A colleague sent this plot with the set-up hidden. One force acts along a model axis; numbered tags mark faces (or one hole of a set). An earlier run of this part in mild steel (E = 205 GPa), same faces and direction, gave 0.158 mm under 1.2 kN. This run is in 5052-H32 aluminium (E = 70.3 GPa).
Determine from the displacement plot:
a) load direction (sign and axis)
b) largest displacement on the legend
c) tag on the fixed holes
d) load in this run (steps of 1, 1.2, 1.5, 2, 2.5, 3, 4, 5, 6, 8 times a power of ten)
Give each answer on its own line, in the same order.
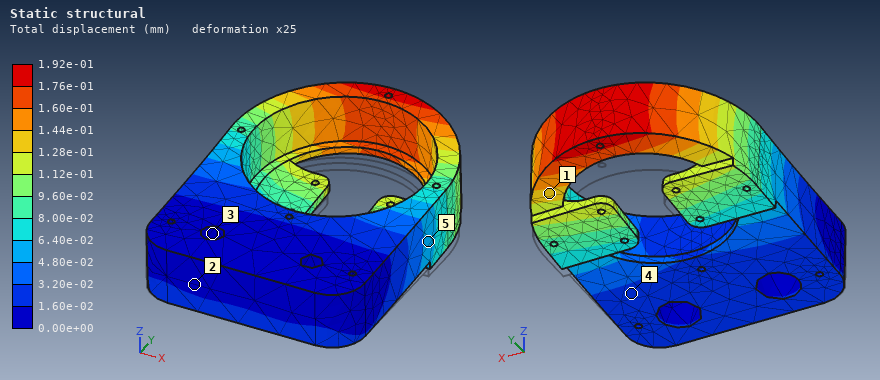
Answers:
+Z
1.92e-01 mm
3
500 N
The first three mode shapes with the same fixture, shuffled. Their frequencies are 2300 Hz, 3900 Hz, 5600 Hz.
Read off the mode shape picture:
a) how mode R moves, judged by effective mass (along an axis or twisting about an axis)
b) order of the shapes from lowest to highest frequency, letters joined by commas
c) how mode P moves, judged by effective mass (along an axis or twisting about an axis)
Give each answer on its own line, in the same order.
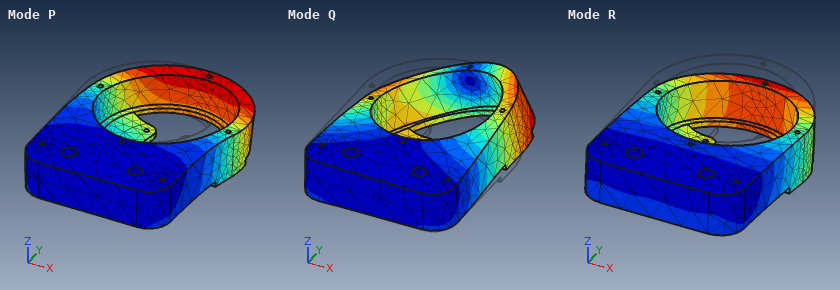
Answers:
along Z
R, P, Q
along X
